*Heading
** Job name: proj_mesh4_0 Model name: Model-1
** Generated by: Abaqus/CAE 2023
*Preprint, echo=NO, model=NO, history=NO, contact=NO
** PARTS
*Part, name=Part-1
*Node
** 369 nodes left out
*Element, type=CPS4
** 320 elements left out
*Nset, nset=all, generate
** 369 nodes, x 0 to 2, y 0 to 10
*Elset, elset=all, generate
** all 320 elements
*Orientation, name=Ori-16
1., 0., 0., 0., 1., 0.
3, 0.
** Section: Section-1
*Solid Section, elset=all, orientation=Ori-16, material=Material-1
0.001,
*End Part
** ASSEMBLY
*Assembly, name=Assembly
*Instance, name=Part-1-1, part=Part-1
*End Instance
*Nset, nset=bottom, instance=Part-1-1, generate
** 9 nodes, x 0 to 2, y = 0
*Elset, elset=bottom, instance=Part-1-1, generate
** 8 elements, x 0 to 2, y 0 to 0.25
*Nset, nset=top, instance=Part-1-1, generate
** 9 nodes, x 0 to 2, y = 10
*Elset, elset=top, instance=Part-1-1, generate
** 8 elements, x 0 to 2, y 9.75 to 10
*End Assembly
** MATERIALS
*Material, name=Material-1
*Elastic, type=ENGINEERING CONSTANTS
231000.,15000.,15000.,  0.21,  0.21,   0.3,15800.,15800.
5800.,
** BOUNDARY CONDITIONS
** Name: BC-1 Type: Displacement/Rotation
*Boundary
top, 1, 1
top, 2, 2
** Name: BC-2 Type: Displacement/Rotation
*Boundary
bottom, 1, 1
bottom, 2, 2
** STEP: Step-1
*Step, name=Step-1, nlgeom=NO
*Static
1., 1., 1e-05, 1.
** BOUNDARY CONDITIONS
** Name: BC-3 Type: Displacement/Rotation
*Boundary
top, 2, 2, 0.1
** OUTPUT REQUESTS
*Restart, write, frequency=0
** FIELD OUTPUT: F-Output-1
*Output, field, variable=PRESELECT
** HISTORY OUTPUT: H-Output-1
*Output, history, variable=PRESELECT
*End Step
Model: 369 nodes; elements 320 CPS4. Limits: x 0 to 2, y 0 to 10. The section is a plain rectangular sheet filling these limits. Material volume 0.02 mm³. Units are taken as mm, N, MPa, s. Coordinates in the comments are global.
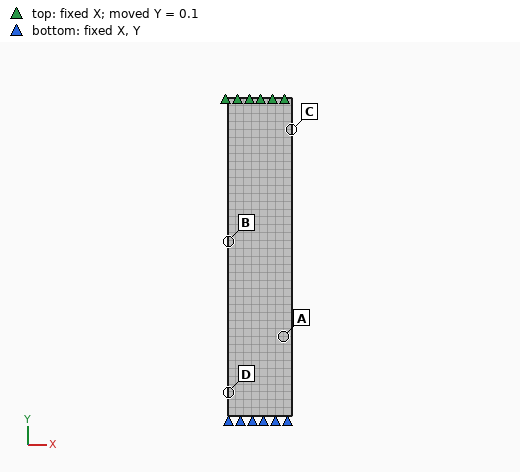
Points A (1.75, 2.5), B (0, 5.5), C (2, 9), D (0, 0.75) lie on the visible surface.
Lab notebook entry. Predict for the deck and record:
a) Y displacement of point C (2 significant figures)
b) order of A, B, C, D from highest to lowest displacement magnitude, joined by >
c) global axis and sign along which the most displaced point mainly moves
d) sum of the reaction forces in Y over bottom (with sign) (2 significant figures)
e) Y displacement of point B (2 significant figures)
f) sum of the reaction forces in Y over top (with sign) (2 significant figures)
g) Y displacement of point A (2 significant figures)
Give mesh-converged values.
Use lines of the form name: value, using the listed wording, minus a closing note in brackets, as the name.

Y displacement of point C: 0.090 mm
order of A, B, C, D from highest to lowest displacement magnitude, joined by >: C > B > A > D
global axis and sign along which the most displaced point mainly moves: +Y
sum of the reaction forces in Y over bottom (with sign): -0.30 N
Y displacement of point B: 0.055 mm
sum of the reaction forces in Y over top (with sign): 0.30 N
Y displacement of point A: 0.025 mm
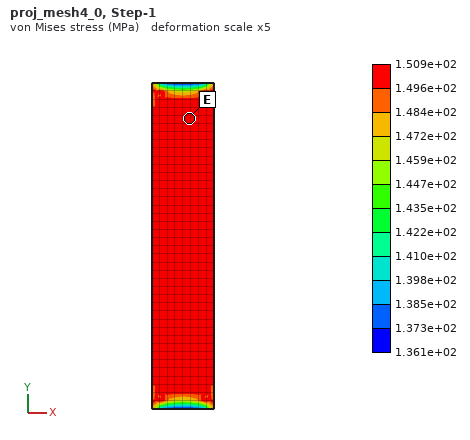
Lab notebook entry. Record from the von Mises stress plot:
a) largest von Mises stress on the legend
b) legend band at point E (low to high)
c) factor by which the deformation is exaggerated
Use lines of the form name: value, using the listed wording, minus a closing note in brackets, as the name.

largest von Mises stress on the legend: 1.509e+02 MPa
legend band at point E: 1.496e+02 to 1.509e+02 MPa
factor by which the deformation is exaggerated: 5
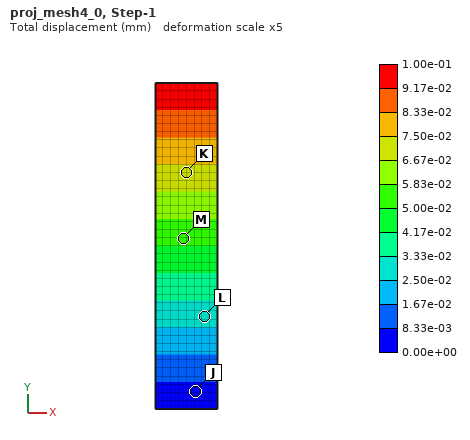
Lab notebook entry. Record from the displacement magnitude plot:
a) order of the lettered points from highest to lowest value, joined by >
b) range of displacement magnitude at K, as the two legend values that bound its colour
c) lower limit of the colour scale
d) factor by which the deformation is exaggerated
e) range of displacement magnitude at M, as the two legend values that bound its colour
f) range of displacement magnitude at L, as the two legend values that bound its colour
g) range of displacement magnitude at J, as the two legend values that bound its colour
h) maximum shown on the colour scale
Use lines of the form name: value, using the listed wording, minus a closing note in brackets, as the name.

order of the lettered points from highest to lowest value, joined by >: K > M > L > J
range of displacement magnitude at K, as the two legend values that bound its colour: 6.67e-02 to 7.50e-02 mm
lower limit of the colour scale: 0.00e+00 mm
factor by which the deformation is exaggerated: 5
range of displacement magnitude at M, as the two legend values that bound its colour: 5.00e-02 to 5.83e-02 mm
range of displacement magnitude at L, as the two legend values that bound its colour: 2.50e-02 to 3.33e-02 mm
range of displacement magnitude at J, as the two legend values that bound its colour: 0.00e+00 to 8.33e-03 mm
maximum shown on the colour scale: 1.00e-01 mm
